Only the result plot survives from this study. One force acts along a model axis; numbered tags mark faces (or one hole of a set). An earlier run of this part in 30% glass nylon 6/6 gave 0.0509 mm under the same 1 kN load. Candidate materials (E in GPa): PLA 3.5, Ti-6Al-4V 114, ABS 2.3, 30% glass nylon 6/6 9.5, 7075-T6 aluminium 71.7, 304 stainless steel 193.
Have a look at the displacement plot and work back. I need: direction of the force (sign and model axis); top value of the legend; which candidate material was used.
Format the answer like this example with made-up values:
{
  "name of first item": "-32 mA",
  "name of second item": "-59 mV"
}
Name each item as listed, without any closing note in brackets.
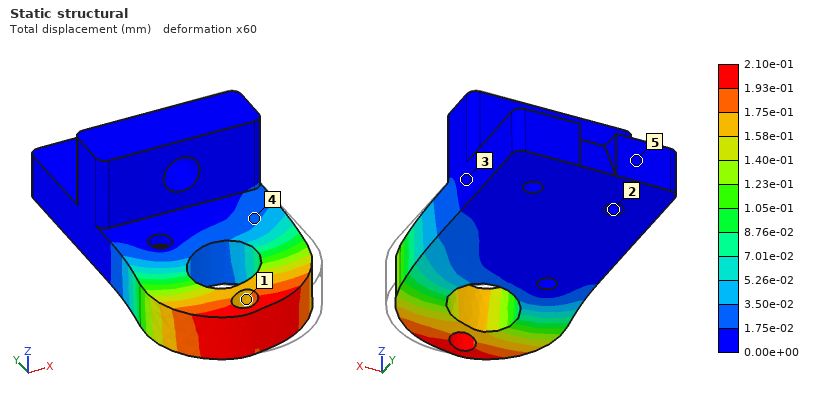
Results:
{
  "direction of the force": "-X",
  "top value of the legend": "2.10e-01 mm",
  "which candidate material was used": "ABS"
}
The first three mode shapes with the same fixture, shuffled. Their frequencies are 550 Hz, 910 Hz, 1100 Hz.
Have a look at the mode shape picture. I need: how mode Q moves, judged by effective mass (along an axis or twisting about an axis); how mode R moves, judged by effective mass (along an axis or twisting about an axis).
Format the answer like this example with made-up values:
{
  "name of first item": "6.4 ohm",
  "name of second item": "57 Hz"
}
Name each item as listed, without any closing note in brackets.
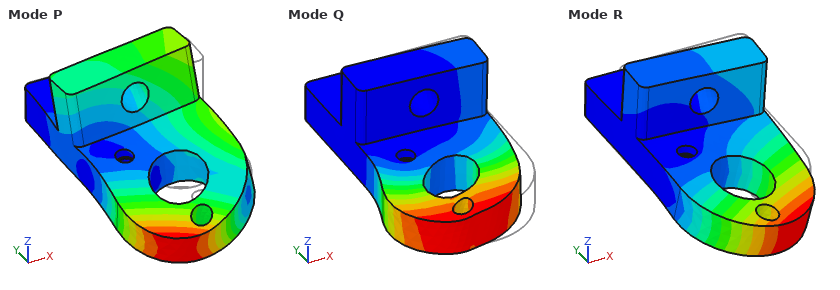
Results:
{
  "how mode Q moves, judged by effective mass": "along X",
  "how mode R moves, judged by effective mass": "along Z"
}
